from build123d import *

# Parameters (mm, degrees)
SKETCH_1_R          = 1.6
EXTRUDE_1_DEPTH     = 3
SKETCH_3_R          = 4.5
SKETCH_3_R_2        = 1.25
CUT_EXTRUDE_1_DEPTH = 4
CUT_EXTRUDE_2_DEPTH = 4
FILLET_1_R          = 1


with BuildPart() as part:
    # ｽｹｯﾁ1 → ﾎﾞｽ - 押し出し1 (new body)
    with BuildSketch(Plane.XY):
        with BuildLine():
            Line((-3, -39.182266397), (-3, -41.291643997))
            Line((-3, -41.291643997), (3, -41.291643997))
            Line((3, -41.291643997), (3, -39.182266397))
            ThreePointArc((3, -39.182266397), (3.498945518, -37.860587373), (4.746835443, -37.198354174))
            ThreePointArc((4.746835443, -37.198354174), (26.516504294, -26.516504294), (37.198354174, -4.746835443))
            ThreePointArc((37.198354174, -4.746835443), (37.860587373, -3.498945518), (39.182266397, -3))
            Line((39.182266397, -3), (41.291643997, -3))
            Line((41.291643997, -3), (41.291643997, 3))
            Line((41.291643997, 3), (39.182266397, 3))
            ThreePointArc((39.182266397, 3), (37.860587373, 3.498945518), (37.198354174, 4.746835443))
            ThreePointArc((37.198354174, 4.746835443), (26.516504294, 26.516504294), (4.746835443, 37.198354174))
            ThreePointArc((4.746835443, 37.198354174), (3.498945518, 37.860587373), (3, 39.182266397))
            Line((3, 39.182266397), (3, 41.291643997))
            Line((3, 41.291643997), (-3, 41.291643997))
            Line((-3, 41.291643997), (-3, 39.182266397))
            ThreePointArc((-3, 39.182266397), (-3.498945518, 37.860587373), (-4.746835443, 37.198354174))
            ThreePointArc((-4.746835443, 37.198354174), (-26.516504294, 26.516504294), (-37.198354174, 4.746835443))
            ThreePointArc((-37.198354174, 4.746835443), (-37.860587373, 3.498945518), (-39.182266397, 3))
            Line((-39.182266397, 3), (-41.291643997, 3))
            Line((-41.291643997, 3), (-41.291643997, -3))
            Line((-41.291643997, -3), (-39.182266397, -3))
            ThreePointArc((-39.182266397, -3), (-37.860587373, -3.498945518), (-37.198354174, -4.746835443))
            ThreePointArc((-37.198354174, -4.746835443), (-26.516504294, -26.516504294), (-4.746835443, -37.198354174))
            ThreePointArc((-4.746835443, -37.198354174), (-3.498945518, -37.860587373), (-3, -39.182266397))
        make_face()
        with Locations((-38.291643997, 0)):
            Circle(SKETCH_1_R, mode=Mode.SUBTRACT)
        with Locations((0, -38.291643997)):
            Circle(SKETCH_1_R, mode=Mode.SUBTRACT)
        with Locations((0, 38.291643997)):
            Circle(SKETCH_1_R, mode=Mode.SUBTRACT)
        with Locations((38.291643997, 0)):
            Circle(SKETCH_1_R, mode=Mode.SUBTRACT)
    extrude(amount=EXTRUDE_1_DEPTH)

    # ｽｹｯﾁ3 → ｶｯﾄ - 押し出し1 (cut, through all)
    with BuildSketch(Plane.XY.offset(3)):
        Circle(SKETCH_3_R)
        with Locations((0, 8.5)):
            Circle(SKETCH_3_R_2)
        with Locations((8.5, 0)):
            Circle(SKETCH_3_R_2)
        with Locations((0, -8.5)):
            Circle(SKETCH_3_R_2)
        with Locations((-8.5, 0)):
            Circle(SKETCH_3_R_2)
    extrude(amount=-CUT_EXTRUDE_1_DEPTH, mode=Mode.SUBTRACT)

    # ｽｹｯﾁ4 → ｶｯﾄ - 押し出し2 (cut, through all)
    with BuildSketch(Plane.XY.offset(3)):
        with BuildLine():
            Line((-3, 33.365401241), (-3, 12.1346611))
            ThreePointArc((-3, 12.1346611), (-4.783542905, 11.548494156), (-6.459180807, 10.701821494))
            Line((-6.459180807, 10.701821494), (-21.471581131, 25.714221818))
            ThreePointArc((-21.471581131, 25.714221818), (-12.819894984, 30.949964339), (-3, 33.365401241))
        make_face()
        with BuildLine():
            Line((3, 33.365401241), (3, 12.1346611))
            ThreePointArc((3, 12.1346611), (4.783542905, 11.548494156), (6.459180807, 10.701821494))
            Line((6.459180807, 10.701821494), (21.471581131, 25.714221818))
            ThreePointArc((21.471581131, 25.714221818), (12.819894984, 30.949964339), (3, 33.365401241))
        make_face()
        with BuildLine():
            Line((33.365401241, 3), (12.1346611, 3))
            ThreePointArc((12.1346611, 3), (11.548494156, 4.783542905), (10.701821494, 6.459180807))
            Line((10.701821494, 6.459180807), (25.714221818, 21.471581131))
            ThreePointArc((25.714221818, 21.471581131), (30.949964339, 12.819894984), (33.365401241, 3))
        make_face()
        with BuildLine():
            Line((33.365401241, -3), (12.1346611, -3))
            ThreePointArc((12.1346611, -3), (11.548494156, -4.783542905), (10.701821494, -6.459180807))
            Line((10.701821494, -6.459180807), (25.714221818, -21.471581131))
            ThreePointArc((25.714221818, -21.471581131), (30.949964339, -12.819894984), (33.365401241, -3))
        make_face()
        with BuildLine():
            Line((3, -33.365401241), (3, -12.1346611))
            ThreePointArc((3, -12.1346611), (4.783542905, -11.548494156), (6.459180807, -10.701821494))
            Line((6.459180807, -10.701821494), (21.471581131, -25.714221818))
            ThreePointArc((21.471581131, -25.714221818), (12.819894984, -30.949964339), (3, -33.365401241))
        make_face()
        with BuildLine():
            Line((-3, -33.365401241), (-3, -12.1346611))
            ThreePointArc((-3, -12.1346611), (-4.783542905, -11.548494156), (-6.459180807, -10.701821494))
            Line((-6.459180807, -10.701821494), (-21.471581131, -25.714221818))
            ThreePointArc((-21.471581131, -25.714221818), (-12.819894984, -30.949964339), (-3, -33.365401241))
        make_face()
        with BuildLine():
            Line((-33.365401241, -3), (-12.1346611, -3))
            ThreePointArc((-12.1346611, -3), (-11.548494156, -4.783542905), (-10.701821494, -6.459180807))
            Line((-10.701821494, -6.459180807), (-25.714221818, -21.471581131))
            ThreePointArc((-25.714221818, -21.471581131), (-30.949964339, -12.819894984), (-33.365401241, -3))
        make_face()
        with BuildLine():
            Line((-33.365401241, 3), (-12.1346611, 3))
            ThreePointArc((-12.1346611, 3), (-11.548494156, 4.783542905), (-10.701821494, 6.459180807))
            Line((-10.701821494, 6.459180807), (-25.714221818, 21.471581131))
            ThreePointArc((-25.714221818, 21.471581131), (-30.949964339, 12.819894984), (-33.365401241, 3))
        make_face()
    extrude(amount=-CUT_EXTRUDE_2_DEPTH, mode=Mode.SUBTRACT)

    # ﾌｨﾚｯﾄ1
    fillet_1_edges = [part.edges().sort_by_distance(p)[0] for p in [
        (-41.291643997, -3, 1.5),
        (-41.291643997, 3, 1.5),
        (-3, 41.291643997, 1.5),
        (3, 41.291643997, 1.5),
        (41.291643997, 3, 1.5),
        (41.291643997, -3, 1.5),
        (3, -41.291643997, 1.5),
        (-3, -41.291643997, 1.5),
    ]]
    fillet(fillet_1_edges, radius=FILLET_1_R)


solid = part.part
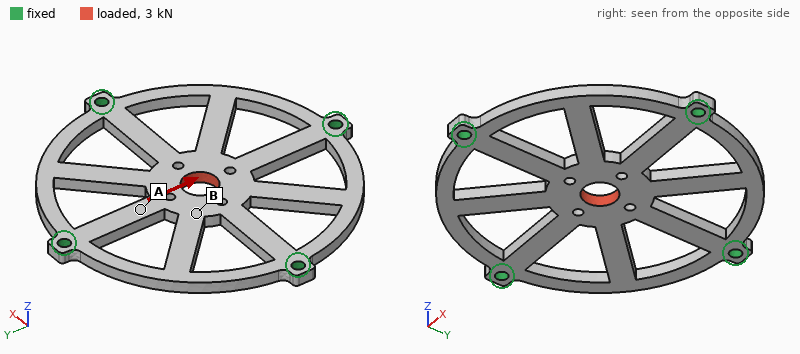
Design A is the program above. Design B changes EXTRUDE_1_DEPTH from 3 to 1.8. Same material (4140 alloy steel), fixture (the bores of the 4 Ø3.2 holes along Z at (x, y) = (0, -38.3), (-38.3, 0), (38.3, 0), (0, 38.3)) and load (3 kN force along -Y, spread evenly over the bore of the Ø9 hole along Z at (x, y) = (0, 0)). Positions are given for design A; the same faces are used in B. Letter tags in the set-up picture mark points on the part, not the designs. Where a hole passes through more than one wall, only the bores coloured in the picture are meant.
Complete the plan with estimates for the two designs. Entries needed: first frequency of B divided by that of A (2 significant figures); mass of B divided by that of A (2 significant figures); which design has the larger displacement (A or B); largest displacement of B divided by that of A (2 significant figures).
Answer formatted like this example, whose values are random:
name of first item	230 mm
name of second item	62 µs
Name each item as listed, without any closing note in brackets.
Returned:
first frequency of B divided by that of A	0.62
mass of B divided by that of A	0.60
which design has the larger displacement	B
largest displacement of B divided by that of A	1.7
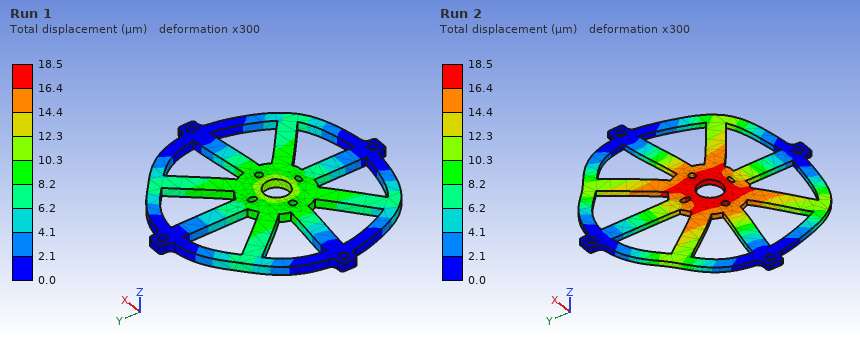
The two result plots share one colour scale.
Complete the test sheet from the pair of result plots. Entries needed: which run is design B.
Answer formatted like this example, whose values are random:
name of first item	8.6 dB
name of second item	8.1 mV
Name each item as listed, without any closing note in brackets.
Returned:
which run is design B	Run 2
